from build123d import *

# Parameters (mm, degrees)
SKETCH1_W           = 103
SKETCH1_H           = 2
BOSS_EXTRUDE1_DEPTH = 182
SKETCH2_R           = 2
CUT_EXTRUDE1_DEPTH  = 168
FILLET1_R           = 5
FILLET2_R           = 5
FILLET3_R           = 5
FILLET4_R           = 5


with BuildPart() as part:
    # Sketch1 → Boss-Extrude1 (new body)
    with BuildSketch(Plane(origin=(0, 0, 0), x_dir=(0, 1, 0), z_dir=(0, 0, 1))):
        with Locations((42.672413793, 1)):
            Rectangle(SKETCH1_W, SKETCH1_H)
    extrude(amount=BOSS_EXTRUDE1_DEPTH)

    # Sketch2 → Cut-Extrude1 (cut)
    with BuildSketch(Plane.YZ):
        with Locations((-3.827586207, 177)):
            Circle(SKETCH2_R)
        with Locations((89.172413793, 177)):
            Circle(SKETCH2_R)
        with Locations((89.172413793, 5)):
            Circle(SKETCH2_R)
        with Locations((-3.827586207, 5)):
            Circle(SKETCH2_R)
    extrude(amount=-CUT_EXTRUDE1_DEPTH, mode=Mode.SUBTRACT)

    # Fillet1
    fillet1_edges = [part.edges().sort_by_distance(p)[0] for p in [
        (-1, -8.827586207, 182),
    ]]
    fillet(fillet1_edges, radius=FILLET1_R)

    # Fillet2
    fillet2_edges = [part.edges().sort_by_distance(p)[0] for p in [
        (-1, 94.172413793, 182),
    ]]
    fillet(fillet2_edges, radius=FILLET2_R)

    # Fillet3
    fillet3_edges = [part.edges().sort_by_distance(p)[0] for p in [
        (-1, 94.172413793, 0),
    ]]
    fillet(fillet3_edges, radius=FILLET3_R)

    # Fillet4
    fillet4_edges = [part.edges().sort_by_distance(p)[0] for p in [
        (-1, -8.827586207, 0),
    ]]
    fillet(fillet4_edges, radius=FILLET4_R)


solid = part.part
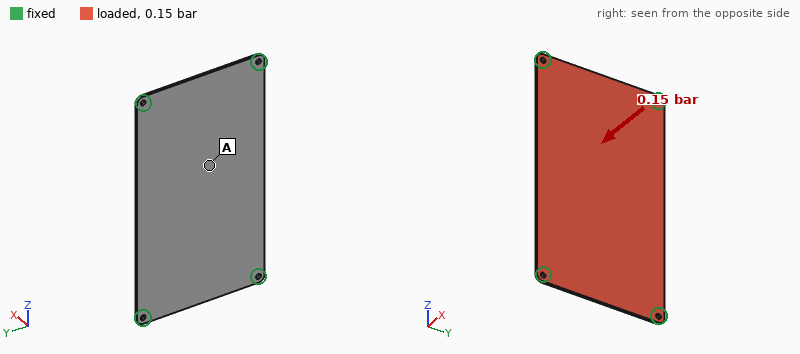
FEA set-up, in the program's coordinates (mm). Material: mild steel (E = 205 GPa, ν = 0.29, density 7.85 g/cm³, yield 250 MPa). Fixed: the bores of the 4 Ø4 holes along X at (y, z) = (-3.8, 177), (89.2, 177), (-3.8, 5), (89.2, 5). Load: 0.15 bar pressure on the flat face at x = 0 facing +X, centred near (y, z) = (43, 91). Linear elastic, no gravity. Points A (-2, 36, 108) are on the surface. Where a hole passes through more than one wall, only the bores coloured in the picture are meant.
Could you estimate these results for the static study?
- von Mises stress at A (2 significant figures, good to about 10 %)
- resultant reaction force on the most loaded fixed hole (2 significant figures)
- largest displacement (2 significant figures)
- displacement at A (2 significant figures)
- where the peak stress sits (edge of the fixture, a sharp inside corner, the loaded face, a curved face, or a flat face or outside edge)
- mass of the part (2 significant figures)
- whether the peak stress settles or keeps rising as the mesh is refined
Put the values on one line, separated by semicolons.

28 MPa; 70 N; 0.39 mm; 0.37 mm; edge of the fixture; 290 g; keeps rising
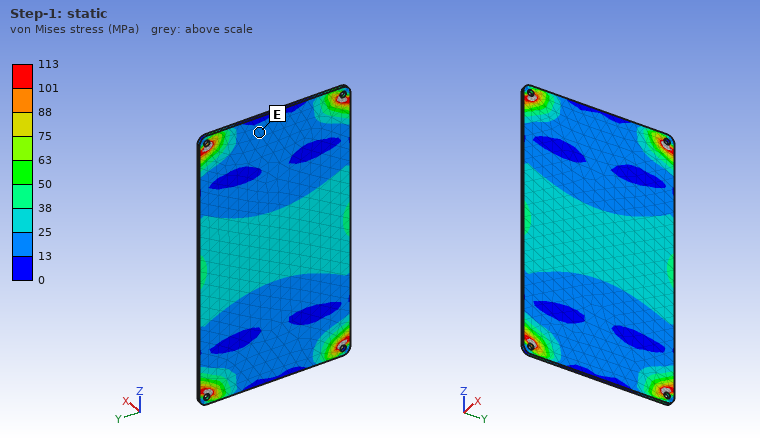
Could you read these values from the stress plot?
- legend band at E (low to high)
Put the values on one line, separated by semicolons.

13 to 25 MPa
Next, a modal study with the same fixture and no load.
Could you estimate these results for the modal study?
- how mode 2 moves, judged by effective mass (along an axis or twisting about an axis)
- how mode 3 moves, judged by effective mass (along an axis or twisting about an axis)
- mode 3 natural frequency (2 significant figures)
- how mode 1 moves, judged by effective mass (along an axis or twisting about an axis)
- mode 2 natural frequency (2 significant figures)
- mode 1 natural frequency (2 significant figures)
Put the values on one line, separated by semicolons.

twisting about Z; twisting about Y; 780 Hz; along X; 520 Hz; 280 Hz
